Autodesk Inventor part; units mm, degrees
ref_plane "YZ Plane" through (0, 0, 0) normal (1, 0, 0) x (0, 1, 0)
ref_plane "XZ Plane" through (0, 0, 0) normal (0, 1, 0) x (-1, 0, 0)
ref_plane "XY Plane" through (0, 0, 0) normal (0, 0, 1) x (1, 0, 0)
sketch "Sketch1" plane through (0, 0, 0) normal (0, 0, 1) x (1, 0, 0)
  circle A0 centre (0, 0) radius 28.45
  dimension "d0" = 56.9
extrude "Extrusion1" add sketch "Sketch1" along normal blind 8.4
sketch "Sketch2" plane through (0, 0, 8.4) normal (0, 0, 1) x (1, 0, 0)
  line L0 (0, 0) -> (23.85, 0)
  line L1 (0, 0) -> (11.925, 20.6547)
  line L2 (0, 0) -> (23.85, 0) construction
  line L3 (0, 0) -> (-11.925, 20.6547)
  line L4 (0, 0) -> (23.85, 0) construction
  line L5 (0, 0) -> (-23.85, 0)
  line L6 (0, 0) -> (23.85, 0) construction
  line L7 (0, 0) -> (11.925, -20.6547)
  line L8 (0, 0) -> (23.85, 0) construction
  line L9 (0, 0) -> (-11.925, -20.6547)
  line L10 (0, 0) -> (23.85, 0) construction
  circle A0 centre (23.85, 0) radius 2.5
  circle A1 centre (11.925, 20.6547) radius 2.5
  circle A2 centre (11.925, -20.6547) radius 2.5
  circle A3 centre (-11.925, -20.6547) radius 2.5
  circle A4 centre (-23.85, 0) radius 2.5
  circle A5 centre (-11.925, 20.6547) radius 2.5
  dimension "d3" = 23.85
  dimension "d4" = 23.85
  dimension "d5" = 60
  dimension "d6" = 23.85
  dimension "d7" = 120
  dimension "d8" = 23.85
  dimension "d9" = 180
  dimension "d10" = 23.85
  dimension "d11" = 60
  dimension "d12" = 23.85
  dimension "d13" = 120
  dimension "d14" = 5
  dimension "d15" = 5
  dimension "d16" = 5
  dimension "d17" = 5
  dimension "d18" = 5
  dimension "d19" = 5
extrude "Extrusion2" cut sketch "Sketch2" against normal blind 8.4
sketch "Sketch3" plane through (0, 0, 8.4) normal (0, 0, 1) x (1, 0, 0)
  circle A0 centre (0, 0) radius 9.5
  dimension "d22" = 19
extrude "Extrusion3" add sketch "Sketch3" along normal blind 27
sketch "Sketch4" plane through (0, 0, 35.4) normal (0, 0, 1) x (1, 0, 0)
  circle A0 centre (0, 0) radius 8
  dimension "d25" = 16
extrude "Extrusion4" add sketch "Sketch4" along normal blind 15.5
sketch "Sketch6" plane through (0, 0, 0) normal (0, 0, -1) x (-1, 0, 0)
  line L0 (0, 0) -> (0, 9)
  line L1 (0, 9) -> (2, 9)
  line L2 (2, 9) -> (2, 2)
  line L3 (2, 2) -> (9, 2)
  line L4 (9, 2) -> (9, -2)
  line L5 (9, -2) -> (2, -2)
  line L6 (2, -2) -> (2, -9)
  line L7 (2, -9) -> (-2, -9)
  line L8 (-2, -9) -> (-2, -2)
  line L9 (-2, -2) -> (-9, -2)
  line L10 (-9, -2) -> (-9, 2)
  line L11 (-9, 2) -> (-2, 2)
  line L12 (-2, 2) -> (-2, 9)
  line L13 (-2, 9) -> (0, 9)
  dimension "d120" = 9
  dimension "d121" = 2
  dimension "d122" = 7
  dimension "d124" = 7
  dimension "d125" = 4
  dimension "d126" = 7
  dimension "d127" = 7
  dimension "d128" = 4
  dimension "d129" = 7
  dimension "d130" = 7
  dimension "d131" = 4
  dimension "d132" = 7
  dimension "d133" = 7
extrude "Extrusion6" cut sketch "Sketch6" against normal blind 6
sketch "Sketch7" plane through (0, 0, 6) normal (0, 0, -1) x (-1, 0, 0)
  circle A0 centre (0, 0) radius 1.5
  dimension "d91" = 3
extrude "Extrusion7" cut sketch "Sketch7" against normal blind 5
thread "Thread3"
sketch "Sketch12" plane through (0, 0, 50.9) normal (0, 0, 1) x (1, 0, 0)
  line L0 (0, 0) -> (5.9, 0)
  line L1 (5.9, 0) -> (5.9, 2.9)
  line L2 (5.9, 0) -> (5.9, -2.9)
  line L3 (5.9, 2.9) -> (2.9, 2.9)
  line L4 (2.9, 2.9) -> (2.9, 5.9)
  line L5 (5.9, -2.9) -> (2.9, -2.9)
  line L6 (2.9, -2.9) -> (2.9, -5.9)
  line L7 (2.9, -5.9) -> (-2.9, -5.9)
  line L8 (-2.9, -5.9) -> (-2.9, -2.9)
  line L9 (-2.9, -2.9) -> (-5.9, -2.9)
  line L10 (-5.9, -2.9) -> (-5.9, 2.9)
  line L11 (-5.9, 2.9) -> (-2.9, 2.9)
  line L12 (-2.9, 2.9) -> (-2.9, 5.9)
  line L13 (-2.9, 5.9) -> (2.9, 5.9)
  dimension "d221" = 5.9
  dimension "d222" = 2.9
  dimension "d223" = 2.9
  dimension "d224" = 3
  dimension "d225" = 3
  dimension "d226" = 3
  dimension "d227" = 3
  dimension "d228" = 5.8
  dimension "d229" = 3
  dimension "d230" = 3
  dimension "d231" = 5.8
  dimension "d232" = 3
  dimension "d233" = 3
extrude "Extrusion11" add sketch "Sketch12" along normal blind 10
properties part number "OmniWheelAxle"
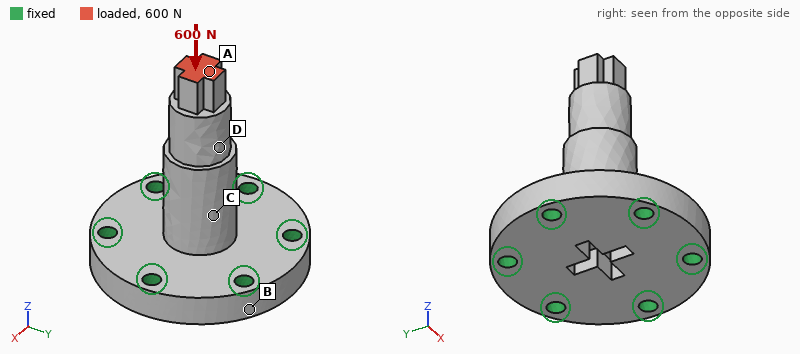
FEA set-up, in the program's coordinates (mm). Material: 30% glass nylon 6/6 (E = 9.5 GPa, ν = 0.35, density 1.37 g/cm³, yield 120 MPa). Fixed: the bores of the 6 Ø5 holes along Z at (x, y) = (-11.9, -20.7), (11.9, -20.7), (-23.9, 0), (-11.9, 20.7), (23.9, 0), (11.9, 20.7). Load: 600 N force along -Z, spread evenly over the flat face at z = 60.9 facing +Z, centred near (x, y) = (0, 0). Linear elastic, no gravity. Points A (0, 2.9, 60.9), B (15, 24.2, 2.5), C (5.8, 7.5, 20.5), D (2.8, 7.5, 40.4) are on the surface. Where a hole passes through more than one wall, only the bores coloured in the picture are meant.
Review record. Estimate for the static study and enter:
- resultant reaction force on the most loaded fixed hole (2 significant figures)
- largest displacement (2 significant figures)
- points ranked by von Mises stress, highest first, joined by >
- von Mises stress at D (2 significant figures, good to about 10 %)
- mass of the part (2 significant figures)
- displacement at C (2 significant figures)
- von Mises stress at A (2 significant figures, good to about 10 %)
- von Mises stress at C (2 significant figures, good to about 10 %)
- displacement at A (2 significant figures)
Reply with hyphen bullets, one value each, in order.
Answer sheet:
- 120 N
- 29 µm
- A > D > C > B
- 3.1 MPa
- 43 g
- 14 µm
- 5.8 MPa
- 2.1 MPa
- 29 µm
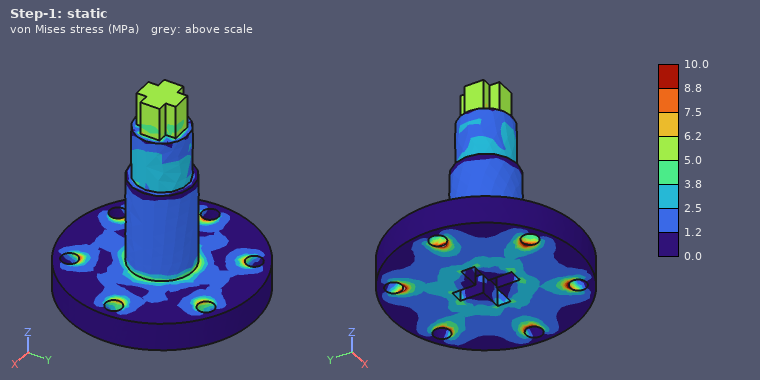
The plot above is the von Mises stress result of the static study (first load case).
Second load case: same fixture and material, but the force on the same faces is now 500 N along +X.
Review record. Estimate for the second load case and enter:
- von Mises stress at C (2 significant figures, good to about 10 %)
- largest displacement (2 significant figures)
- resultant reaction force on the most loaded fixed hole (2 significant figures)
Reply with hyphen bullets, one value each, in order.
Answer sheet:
- 18 MPa
- 0.80 mm
- 540 N
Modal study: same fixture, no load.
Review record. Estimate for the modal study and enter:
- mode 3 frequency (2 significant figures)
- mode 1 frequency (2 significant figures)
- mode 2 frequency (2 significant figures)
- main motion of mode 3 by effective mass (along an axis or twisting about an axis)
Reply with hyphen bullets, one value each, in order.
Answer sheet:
- 7300 Hz
- 2300 Hz
- 2300 Hz
- along Z
